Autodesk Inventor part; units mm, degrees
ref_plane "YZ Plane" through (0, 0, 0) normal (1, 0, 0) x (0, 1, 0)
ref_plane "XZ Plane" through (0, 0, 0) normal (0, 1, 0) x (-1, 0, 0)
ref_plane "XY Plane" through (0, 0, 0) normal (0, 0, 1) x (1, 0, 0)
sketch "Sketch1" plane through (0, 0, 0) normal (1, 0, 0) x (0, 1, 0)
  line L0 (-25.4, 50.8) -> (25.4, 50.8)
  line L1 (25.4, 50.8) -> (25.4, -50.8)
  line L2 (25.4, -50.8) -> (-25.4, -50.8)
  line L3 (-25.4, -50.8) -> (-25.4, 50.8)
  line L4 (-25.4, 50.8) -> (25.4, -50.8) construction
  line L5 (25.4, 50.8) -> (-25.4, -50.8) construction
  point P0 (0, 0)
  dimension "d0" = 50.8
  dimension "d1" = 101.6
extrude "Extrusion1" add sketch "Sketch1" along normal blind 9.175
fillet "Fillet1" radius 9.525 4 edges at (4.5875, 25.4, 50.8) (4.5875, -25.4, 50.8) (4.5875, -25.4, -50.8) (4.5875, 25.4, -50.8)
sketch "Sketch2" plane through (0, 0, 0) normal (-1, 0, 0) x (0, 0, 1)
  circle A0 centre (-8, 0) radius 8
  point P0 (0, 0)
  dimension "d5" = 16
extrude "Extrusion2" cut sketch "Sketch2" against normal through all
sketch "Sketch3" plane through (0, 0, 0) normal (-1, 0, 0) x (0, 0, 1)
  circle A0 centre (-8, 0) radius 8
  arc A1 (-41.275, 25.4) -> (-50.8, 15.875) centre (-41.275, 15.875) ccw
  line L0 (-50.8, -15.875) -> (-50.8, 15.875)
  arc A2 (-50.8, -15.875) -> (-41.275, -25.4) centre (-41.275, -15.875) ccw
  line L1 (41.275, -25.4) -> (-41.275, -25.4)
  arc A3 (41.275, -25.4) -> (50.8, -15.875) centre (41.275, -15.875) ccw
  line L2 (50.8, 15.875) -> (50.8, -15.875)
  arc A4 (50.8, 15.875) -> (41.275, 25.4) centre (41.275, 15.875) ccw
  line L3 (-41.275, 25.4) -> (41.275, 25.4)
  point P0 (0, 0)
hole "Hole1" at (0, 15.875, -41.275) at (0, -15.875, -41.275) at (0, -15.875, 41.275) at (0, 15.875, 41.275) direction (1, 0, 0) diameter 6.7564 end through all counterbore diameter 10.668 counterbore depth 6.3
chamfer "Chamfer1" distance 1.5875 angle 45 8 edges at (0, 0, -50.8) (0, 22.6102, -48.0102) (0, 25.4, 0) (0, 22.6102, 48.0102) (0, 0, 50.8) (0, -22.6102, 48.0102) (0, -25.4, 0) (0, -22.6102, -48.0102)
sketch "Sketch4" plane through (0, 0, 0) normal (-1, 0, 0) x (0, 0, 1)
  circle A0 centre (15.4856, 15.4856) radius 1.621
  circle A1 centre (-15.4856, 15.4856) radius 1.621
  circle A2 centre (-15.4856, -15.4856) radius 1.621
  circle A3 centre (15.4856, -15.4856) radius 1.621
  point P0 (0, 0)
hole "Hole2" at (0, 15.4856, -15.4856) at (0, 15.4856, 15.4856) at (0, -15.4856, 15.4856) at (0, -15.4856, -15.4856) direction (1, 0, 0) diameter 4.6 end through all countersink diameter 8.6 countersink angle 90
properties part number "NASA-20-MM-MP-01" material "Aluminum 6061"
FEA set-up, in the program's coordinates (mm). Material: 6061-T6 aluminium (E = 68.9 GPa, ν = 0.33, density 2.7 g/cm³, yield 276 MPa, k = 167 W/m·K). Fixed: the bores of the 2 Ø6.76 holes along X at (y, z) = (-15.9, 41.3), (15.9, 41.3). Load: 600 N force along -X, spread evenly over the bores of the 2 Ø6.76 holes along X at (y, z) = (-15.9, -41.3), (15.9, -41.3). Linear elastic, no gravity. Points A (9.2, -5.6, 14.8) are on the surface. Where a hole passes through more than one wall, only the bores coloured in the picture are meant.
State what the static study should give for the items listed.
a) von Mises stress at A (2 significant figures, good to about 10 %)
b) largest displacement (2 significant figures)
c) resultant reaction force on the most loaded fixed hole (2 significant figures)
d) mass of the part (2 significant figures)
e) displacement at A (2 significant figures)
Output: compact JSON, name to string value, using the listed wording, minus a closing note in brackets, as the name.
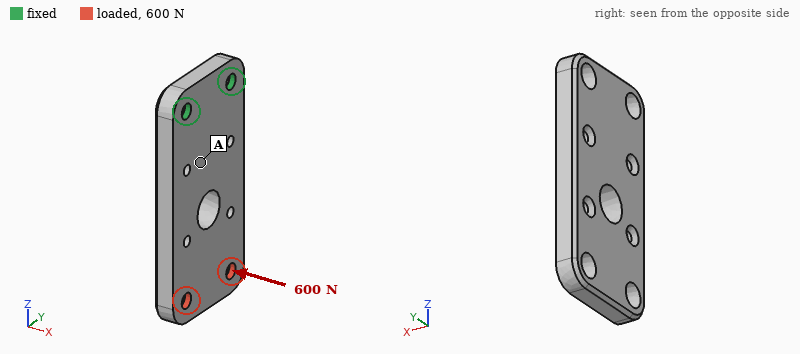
{"von Mises stress at A": "52 MPa", "largest displacement": "1.2 mm", "resultant reaction force on the most loaded fixed hole": "510 N", "mass of the part": "110 g", "displacement at A": "0.21 mm"}
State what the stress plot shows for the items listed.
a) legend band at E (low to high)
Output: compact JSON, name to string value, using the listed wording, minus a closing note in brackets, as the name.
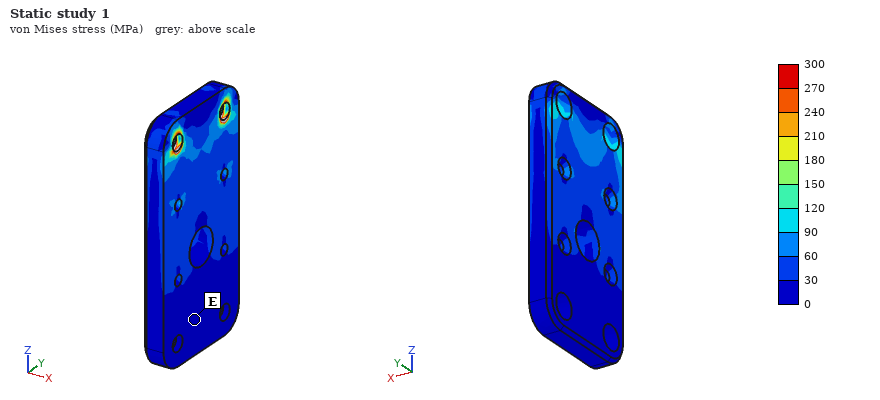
{"legend band at E": "0 to 30 MPa"}
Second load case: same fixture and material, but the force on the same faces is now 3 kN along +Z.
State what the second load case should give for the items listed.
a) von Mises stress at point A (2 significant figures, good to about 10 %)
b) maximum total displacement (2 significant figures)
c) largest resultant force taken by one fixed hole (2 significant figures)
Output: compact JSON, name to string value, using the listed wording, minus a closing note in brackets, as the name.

{"von Mises stress at point A": "19 MPa", "maximum total displacement": "0.19 mm", "largest resultant force taken by one fixed hole": "1.5 kN"}
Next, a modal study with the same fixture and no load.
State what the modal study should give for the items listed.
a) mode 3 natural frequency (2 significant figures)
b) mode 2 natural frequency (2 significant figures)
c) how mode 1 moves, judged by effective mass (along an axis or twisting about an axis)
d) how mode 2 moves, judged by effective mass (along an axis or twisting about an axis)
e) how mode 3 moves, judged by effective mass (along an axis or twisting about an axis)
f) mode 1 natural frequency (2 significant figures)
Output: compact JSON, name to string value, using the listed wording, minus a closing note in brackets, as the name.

{"mode 3 natural frequency": "3500 Hz", "mode 2 natural frequency": "2900 Hz", "how mode 1 moves, judged by effective mass": "along X", "how mode 2 moves, judged by effective mass": "along Y", "how mode 3 moves, judged by effective mass": "along Y", "mode 1 natural frequency": "650 Hz"}
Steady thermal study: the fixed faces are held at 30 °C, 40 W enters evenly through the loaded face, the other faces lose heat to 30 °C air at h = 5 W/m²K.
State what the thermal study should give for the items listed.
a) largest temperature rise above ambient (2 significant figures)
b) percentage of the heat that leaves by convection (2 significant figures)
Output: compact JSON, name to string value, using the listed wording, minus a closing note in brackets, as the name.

{"largest temperature rise above ambient": "60 K", "percentage of the heat that leaves by convection": "4.7 %"}
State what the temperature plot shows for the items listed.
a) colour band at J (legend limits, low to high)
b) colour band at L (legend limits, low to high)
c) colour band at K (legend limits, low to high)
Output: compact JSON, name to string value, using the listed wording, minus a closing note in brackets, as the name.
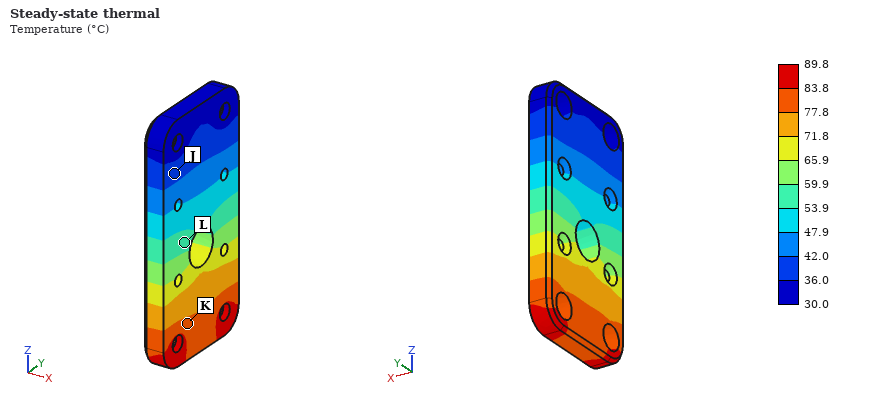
{"colour band at J": "36.0 to 42.0 °C", "colour band at L": "53.9 to 59.9 °C", "colour band at K": "77.8 to 83.8 °C"}
